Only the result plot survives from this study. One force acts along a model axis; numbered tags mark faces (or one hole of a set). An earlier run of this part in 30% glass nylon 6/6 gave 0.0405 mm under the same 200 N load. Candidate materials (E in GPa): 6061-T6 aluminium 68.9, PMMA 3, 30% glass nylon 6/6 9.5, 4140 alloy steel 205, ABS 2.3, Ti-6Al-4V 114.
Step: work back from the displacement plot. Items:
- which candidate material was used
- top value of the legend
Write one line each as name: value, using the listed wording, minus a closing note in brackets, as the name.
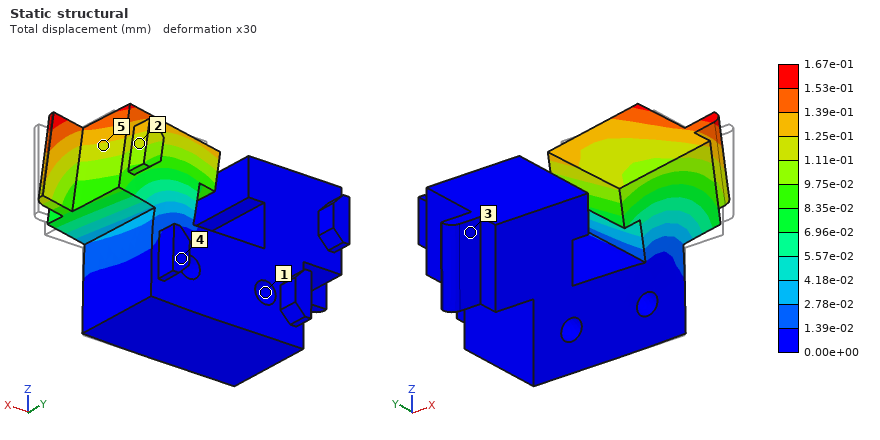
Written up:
which candidate material was used: ABS
top value of the legend: 1.67e-01 mm
